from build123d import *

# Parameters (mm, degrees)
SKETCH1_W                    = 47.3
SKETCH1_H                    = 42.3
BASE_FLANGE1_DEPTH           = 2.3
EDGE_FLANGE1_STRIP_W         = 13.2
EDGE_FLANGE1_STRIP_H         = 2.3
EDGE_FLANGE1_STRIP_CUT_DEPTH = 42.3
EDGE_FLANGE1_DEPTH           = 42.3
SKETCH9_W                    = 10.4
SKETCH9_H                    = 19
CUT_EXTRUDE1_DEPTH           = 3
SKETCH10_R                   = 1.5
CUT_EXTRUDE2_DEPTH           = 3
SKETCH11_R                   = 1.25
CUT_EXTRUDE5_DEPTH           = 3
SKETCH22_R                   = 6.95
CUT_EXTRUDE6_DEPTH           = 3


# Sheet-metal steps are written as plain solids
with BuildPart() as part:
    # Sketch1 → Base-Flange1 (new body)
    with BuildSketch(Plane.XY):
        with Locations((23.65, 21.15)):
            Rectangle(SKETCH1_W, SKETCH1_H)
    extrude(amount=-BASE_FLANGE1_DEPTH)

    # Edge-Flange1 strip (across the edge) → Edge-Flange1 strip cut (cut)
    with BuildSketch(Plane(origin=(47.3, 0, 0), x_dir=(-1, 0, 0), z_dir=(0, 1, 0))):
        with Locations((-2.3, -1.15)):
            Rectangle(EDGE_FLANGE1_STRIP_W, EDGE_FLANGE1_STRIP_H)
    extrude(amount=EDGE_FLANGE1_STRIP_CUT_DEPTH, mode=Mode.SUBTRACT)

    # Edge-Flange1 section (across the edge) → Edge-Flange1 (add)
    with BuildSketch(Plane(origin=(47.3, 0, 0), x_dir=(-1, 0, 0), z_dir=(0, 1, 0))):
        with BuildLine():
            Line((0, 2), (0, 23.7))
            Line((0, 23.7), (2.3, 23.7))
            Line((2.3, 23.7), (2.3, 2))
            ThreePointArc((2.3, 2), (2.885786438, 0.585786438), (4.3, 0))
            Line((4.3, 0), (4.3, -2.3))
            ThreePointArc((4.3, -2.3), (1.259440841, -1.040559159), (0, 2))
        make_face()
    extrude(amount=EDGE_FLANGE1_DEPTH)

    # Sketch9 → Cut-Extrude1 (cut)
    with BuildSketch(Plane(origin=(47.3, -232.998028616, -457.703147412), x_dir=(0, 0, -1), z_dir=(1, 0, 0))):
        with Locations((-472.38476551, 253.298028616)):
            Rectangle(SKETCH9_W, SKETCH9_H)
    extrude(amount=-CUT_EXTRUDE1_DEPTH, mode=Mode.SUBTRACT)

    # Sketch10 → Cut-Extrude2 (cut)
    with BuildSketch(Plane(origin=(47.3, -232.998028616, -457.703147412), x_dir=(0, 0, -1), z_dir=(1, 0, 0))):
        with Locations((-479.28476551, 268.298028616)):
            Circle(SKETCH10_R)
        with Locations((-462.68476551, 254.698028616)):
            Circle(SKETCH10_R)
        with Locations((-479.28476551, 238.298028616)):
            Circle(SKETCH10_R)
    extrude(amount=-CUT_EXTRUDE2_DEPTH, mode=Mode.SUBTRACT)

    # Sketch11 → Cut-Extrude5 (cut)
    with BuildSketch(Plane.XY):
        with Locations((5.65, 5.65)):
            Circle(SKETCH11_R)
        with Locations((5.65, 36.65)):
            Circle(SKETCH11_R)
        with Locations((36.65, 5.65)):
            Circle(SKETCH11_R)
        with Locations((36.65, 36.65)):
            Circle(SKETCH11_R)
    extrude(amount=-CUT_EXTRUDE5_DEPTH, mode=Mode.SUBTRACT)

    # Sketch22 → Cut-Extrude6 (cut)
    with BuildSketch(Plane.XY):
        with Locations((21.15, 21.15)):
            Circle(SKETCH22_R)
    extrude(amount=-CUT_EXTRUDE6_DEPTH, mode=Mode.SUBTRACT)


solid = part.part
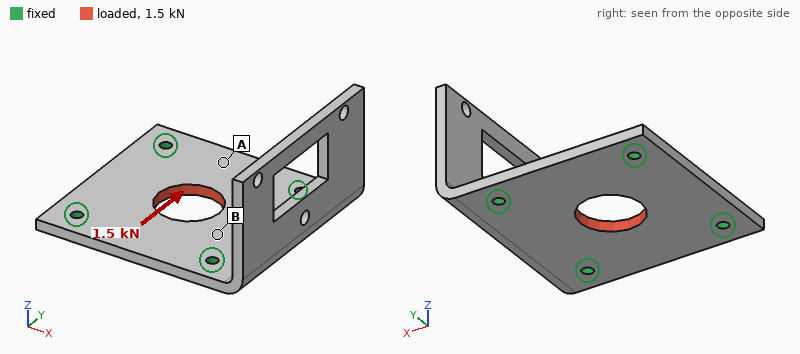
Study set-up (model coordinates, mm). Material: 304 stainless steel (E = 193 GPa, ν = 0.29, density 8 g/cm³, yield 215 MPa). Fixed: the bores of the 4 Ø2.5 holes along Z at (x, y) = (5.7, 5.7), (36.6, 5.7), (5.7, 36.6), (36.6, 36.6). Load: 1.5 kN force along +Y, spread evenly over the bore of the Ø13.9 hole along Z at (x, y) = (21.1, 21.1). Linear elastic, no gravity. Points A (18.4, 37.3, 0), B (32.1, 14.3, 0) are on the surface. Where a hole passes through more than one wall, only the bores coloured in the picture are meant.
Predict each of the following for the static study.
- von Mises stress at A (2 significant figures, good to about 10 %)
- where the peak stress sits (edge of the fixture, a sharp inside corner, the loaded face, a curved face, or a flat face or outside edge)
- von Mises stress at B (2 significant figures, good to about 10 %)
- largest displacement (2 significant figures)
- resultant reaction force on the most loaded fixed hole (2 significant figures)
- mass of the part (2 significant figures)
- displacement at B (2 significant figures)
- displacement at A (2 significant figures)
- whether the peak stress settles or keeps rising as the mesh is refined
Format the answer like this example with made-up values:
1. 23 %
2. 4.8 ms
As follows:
1. 6.4 MPa
2. edge of the fixture
3. 15 MPa
4. 2.1 µm
5. 410 N
6. 47 g
7. 0.92 µm
8. 1.6 µm
9. keeps rising
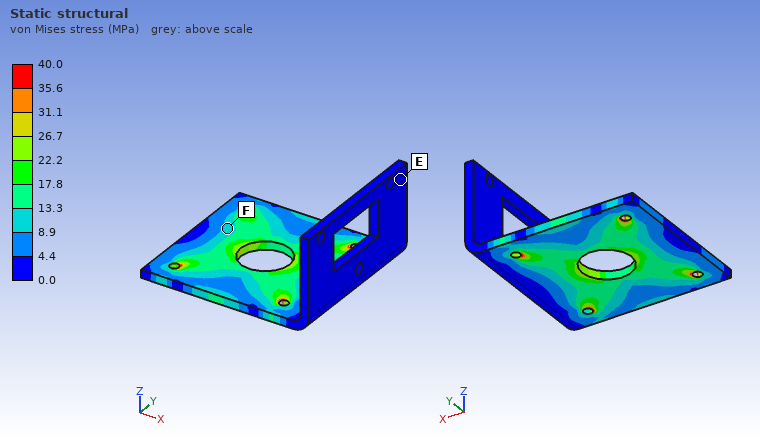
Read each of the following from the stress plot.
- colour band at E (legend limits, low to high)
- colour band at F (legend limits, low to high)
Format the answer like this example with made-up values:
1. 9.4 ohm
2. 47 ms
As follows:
1. 0.0 to 4.4 MPa
2. 8.9 to 13.3 MPa
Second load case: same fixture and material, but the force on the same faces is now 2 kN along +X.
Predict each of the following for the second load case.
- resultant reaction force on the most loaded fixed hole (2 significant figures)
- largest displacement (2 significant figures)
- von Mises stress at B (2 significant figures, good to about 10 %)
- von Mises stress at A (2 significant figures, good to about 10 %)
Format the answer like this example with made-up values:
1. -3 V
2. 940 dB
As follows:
1. 540 N
2. 2.8 µm
3. 17 MPa
4. 8.3 MPa
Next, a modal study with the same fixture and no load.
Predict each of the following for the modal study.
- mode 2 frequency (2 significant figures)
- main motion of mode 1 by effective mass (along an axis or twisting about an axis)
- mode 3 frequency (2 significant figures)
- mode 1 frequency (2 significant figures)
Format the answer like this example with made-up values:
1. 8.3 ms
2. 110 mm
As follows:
1. 3500 Hz
2. along X
3. 6600 Hz
4. 2000 Hz
